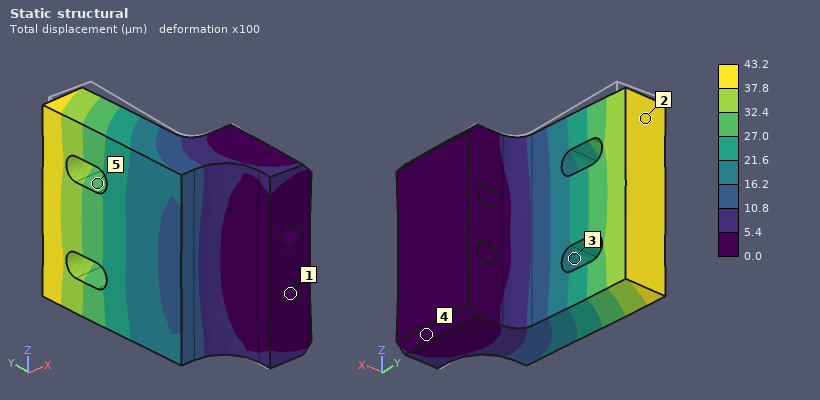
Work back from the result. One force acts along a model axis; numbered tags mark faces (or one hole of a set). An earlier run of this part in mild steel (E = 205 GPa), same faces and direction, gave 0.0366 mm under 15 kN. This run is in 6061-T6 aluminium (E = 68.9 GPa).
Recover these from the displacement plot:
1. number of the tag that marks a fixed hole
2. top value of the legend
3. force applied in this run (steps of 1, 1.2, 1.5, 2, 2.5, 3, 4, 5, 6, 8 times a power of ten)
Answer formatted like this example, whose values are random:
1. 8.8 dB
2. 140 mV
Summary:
1. 1
2. 43.2 µm
3. 6 kN
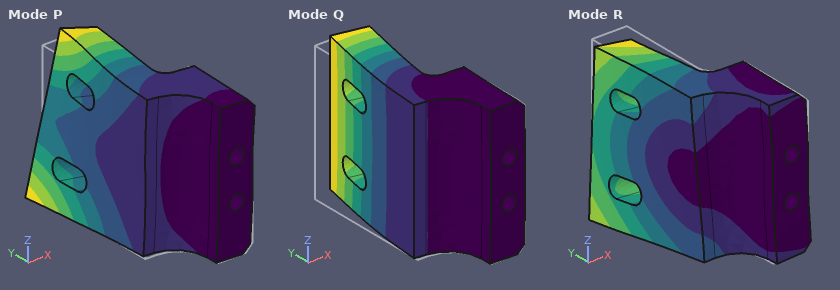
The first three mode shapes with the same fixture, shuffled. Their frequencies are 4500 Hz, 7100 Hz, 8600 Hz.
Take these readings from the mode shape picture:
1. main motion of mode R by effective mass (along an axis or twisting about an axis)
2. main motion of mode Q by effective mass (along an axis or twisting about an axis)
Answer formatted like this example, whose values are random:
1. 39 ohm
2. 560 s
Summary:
1. along Z
2. along X
